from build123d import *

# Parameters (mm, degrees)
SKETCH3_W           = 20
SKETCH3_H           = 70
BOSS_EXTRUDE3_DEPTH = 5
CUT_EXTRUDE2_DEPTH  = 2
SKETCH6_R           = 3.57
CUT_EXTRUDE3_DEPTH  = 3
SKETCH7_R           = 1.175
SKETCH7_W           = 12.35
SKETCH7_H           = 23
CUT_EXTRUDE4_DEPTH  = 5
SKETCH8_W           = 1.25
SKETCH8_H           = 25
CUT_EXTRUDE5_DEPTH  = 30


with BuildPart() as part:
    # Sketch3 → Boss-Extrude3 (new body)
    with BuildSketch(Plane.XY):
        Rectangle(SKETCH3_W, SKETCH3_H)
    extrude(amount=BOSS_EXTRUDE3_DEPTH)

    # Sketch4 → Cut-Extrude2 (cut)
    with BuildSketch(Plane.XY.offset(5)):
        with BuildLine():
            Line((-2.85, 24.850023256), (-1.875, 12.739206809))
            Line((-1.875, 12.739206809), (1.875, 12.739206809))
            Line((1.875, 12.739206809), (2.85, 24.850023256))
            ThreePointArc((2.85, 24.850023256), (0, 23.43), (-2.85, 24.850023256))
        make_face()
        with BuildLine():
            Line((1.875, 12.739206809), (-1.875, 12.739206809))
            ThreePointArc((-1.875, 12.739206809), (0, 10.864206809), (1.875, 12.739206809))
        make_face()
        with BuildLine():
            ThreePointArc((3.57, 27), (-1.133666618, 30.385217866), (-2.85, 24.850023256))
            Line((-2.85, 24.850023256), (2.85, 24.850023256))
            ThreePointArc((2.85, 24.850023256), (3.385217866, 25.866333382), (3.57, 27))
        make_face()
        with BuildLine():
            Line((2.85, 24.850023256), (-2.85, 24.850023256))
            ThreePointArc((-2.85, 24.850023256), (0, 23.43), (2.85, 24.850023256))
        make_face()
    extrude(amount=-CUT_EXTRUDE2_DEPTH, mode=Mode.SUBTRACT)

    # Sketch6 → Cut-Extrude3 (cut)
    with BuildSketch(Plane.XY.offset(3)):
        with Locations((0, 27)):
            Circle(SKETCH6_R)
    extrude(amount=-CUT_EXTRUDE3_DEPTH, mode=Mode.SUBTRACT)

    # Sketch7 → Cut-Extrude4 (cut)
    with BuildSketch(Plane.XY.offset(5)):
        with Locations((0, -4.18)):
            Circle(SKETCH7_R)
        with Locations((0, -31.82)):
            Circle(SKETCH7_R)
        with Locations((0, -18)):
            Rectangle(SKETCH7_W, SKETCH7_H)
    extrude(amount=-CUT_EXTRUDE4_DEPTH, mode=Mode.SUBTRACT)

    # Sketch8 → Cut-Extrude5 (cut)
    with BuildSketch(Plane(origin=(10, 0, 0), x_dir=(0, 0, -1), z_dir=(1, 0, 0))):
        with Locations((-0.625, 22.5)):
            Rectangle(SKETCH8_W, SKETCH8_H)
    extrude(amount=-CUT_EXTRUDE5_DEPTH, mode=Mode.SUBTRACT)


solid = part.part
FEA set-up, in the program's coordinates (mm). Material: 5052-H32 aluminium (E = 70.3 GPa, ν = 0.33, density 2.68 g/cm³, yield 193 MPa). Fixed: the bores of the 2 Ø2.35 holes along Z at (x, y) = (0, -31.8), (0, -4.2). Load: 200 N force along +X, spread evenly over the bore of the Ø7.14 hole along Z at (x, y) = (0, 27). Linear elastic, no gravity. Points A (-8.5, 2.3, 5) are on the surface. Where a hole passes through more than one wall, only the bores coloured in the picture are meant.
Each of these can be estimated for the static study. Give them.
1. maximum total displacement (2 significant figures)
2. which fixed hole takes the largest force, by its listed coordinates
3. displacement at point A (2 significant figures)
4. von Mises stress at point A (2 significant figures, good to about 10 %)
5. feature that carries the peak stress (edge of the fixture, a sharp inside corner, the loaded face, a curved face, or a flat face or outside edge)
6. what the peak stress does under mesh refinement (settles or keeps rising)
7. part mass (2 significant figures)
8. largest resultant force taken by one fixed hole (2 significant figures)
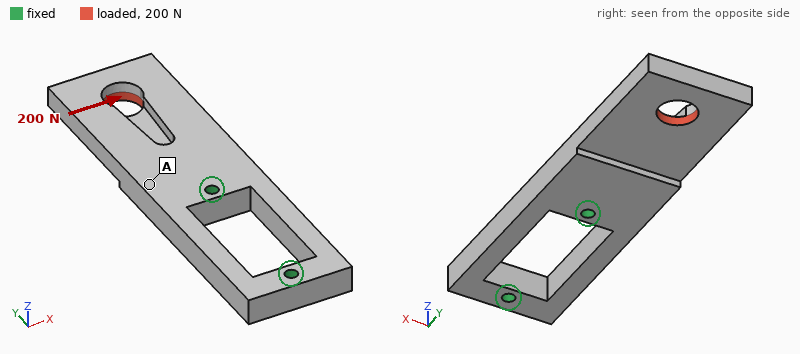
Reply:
72 µm
(0, -4.2)
15 µm
14 MPa
edge of the fixture
keeps rising
12 g
260 N
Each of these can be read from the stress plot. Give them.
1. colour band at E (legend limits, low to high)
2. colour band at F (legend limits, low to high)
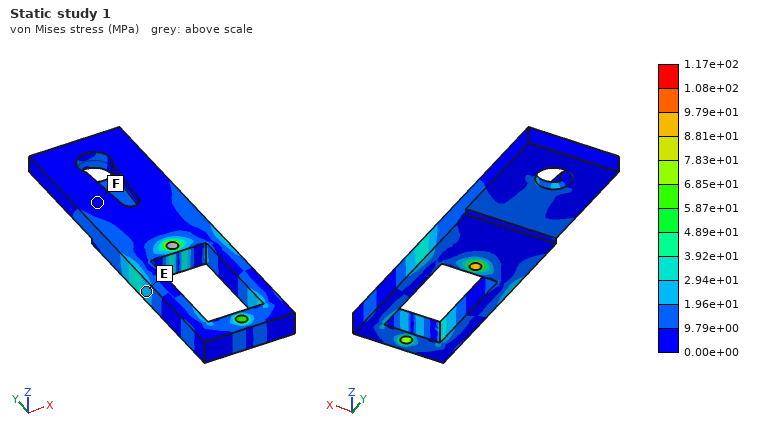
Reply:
1.96e+01 to 2.94e+01 MPa
0.00e+00 to 9.79e+00 MPa
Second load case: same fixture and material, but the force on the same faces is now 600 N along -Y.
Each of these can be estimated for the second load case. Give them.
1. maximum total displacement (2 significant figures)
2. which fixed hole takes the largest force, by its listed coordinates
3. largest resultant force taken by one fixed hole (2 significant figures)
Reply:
40 µm
(0, -4.2)
550 N
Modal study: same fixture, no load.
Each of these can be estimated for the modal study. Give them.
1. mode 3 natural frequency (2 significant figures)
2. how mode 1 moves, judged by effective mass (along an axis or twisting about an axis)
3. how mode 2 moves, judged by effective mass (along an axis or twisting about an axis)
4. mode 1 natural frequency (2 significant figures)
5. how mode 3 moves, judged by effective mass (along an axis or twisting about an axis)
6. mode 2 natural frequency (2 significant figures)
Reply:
7600 Hz
along Z
along X
2700 Hz
twisting about Y
4900 Hz
